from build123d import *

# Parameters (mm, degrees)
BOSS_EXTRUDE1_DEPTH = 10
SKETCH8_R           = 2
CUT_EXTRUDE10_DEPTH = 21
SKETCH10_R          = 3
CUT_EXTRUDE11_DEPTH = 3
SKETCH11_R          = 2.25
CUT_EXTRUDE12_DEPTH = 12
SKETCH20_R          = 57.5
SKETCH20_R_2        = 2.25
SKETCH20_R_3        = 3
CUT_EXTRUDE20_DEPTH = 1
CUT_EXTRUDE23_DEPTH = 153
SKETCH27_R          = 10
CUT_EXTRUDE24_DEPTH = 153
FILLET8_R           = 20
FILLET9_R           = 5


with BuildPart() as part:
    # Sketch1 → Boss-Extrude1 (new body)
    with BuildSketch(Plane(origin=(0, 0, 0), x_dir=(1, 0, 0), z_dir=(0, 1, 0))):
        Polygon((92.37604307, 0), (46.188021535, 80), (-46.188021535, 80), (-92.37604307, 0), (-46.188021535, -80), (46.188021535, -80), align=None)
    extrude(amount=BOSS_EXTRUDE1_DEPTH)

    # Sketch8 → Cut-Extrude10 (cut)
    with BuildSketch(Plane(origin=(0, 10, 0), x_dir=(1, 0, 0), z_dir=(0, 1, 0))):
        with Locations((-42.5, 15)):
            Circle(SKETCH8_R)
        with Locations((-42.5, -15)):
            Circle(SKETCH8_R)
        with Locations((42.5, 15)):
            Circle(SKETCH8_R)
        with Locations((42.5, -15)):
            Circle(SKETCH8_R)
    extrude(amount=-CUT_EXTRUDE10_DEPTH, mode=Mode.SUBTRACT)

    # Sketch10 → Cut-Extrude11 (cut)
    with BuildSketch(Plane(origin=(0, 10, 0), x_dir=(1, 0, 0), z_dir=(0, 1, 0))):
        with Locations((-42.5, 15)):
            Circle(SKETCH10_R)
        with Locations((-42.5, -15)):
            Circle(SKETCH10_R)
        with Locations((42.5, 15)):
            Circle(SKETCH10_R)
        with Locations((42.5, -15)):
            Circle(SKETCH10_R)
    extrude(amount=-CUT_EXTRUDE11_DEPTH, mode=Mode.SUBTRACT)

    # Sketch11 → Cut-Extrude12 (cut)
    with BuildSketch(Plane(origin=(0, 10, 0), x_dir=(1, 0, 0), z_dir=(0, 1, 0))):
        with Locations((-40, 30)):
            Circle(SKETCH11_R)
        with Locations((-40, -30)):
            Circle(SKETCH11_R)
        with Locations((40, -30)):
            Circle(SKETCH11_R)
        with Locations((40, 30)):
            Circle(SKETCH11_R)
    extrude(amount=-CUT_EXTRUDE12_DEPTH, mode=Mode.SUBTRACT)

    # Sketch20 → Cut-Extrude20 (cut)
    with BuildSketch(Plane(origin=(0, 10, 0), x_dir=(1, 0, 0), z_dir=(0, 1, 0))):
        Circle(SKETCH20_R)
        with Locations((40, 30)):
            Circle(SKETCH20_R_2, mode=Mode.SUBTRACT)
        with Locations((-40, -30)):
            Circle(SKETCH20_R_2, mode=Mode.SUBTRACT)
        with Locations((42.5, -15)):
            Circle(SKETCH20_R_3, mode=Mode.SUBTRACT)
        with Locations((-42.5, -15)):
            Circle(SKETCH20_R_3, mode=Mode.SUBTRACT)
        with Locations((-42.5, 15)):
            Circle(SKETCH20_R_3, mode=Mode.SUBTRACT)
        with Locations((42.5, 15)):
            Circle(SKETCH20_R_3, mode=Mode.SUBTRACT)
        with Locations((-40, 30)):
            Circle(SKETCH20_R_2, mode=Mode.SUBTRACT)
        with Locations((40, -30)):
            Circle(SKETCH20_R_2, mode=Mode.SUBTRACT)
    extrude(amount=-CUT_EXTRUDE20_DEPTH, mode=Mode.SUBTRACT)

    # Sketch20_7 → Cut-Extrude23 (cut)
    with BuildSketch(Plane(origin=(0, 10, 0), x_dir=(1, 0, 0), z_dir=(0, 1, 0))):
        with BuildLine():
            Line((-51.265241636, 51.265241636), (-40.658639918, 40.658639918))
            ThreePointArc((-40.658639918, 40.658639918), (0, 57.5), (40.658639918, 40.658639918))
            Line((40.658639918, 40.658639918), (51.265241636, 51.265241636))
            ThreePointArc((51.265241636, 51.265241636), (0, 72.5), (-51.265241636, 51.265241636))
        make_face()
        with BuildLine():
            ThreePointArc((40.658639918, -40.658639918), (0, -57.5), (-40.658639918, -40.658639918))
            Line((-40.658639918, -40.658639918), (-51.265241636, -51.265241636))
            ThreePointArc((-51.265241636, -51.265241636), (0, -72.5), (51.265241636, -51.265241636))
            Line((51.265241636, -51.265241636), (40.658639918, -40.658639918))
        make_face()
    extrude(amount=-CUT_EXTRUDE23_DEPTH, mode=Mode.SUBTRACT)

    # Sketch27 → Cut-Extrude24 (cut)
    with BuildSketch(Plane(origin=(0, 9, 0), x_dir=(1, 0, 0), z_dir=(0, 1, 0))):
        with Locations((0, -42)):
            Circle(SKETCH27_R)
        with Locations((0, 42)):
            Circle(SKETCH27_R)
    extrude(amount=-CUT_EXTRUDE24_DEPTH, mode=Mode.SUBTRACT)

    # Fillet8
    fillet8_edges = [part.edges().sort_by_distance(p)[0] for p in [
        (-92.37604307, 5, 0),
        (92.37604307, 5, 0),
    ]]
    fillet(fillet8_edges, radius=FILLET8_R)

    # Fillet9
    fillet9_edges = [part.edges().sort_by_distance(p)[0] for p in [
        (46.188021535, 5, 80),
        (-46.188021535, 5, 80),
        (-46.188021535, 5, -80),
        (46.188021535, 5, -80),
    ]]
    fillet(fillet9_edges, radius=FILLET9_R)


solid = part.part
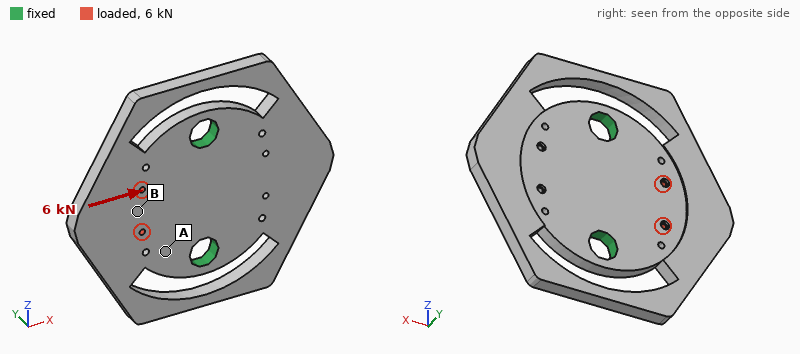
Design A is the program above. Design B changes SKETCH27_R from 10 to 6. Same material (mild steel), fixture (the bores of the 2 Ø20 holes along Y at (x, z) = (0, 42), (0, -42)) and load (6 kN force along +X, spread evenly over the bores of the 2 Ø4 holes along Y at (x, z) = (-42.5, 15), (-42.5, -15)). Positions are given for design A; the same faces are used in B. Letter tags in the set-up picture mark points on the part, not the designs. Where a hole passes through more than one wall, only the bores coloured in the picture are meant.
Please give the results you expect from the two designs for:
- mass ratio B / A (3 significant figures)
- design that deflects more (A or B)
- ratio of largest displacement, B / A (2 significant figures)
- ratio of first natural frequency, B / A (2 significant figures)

1.02
B
1.2
0.85
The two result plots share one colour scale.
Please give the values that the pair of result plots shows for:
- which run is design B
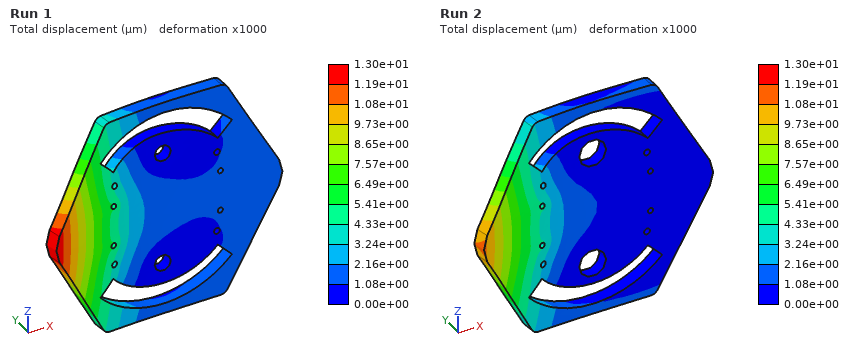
Run 1
